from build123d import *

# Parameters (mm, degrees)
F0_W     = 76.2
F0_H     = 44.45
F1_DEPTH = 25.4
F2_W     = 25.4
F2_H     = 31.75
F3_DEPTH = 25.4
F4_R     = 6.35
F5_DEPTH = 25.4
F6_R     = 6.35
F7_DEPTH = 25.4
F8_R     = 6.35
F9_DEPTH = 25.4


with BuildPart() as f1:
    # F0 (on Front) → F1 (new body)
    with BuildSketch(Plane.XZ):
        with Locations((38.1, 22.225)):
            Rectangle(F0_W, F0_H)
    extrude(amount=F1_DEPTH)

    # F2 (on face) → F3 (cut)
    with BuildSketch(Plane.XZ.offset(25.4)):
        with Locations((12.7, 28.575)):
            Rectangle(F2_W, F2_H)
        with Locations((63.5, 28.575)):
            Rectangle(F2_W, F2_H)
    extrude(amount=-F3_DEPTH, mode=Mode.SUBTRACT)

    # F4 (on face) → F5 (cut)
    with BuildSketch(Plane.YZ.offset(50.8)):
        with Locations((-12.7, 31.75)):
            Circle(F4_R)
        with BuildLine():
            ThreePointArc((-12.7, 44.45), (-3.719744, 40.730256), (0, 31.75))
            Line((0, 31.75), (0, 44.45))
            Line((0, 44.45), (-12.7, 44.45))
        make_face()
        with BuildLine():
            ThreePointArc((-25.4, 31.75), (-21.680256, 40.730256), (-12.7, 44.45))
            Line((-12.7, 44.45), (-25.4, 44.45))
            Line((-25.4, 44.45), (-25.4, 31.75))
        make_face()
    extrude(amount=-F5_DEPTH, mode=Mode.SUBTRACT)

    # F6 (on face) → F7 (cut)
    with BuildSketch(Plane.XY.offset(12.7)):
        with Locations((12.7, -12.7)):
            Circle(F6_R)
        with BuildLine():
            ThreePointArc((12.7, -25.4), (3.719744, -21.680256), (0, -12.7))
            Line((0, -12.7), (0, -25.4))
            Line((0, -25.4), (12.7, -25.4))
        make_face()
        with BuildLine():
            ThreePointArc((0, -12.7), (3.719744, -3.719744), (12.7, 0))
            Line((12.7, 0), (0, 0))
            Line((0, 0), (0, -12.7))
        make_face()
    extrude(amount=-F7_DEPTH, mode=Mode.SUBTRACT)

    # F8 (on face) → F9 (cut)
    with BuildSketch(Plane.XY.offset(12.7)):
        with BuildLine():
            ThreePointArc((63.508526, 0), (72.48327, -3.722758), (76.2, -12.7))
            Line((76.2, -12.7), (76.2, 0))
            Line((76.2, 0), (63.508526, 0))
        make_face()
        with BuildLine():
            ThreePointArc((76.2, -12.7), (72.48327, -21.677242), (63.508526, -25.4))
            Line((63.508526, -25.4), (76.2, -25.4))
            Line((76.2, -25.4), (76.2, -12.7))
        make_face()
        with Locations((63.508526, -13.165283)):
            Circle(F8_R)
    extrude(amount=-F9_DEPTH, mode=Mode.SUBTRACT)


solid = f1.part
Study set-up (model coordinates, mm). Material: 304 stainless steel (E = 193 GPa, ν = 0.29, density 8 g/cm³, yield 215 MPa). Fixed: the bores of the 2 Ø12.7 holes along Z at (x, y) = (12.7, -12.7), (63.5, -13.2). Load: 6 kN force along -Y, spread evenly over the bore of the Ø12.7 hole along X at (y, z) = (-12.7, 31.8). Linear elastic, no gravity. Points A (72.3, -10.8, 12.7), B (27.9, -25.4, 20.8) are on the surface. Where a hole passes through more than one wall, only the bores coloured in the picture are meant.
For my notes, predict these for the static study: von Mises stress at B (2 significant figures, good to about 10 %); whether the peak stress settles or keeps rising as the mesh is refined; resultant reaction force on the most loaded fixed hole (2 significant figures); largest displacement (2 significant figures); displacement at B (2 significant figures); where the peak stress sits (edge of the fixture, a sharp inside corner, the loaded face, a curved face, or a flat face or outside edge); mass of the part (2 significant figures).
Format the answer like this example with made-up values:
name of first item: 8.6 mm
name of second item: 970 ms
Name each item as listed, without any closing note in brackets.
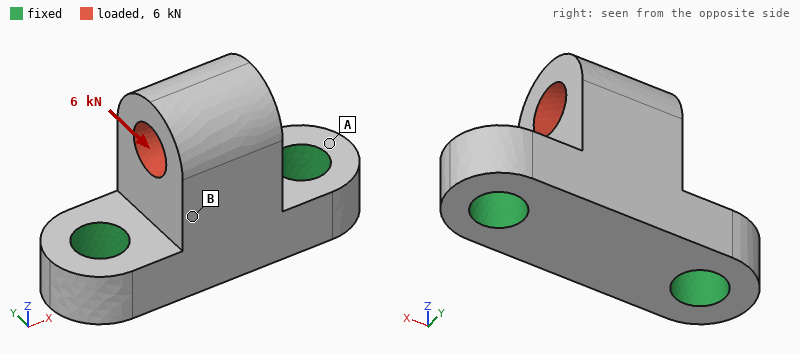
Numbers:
von Mises stress at B: 38 MPa
whether the peak stress settles or keeps rising as the mesh is refined: keeps rising
resultant reaction force on the most loaded fixed hole: 3.0 kN
largest displacement: 47 µm
displacement at B: 21 µm
where the peak stress sits: edge of the fixture
mass of the part: 280 g
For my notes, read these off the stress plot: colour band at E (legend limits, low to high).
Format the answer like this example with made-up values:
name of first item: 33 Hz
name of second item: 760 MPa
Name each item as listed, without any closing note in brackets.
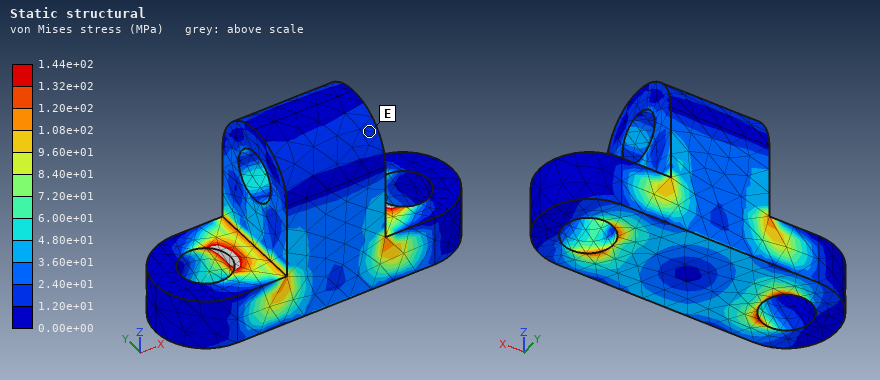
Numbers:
colour band at E: 1.20e+01 to 2.40e+01 MPa
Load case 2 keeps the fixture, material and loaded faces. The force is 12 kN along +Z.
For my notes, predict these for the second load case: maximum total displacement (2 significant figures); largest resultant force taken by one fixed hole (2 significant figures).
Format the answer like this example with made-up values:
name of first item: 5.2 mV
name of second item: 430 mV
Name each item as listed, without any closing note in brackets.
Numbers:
maximum total displacement: 9.8 µm
largest resultant force taken by one fixed hole: 6.2 kN
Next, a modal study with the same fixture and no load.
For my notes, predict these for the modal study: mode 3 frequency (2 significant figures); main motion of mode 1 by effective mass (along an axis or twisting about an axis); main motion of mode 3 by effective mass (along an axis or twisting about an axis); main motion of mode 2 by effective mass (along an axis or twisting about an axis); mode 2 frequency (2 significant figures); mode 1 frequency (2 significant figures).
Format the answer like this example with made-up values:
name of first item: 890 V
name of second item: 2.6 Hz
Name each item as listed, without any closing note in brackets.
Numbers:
mode 3 frequency: 17 kHz
main motion of mode 1 by effective mass: along Y
main motion of mode 3 by effective mass: along Z
main motion of mode 2 by effective mass: along X
mode 2 frequency: 12 kHz
mode 1 frequency: 6800 Hz
